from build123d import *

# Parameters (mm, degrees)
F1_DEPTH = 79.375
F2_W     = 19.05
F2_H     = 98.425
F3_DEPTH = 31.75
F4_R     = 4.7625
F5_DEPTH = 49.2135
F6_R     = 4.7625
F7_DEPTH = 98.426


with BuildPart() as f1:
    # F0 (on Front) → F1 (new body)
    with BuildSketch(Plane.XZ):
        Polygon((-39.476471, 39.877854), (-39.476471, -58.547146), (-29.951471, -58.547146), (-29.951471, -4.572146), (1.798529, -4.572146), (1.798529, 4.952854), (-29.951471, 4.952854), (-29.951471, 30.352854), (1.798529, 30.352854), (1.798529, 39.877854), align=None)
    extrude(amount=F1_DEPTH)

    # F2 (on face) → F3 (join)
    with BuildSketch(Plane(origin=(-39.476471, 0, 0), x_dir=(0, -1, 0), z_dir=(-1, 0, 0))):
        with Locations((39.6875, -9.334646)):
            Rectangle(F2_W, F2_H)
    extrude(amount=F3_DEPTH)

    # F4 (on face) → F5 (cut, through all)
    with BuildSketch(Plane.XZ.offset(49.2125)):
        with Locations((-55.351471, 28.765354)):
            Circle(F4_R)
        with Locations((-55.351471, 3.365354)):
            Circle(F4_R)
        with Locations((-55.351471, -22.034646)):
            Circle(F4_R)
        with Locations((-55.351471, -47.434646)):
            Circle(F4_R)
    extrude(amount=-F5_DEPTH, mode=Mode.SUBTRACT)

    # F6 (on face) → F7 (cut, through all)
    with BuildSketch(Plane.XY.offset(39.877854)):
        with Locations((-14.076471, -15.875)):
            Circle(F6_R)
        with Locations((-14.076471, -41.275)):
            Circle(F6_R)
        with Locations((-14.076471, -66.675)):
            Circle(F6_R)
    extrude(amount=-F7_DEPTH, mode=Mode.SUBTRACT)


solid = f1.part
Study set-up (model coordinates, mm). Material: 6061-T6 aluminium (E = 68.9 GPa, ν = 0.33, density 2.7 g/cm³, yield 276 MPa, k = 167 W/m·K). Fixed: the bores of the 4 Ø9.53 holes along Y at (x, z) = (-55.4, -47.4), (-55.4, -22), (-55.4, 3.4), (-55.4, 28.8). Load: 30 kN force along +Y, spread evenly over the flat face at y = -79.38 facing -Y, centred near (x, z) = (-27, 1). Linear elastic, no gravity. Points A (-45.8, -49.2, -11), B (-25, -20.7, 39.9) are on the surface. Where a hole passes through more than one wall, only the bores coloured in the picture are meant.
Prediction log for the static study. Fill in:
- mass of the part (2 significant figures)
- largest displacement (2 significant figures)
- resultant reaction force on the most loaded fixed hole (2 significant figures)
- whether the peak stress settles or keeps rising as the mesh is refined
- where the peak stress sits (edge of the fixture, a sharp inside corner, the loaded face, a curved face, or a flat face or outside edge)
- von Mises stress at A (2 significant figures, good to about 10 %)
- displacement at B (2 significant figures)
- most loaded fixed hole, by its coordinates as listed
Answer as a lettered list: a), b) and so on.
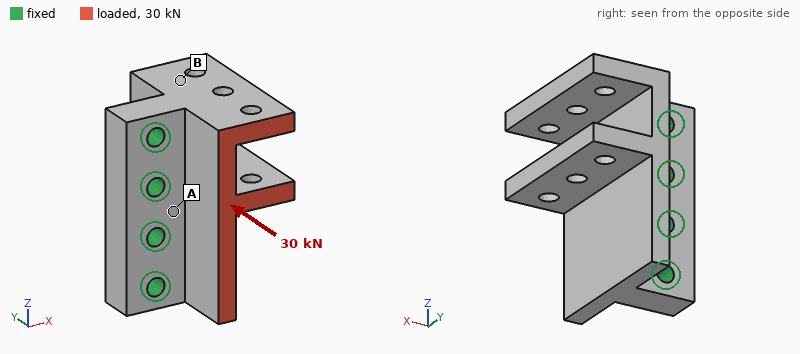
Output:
a) 470 g
b) 0.33 mm
c) 11 kN
d) keeps rising
e) edge of the fixture
f) 72 MPa
g) 0.15 mm
h) (-55.4, 28.8)
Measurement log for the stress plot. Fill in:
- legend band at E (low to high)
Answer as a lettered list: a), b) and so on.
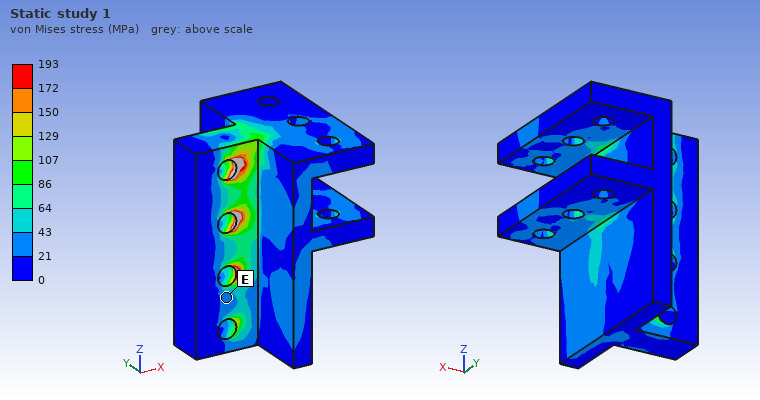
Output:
a) 21 to 43 MPa
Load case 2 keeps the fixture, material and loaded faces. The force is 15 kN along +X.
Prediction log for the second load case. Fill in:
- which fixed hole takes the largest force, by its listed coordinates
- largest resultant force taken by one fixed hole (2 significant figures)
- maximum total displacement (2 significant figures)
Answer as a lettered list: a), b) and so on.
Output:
a) (-55.4, 28.8)
b) 5.6 kN
c) 0.34 mm
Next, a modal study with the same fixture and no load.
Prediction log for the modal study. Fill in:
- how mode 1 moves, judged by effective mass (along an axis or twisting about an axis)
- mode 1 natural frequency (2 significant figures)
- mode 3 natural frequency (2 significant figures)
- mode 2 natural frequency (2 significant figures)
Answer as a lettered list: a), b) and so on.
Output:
a) along Y
b) 3200 Hz
c) 5000 Hz
d) 4500 Hz
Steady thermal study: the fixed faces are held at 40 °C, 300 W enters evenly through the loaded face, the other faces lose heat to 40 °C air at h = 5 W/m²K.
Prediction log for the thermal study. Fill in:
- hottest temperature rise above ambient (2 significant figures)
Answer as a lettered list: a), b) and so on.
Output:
a) 76 K
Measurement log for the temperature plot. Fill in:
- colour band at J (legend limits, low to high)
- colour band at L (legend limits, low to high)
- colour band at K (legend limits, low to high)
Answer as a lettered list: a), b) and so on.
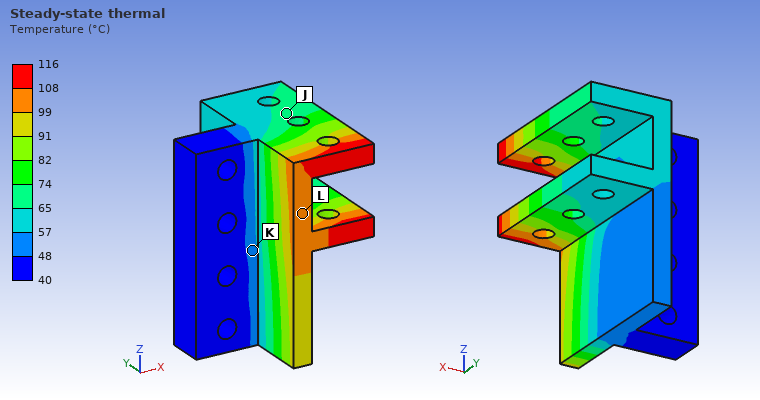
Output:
a) 65 to 74 °C
b) 99 to 108 °C
c) 48 to 57 °C
